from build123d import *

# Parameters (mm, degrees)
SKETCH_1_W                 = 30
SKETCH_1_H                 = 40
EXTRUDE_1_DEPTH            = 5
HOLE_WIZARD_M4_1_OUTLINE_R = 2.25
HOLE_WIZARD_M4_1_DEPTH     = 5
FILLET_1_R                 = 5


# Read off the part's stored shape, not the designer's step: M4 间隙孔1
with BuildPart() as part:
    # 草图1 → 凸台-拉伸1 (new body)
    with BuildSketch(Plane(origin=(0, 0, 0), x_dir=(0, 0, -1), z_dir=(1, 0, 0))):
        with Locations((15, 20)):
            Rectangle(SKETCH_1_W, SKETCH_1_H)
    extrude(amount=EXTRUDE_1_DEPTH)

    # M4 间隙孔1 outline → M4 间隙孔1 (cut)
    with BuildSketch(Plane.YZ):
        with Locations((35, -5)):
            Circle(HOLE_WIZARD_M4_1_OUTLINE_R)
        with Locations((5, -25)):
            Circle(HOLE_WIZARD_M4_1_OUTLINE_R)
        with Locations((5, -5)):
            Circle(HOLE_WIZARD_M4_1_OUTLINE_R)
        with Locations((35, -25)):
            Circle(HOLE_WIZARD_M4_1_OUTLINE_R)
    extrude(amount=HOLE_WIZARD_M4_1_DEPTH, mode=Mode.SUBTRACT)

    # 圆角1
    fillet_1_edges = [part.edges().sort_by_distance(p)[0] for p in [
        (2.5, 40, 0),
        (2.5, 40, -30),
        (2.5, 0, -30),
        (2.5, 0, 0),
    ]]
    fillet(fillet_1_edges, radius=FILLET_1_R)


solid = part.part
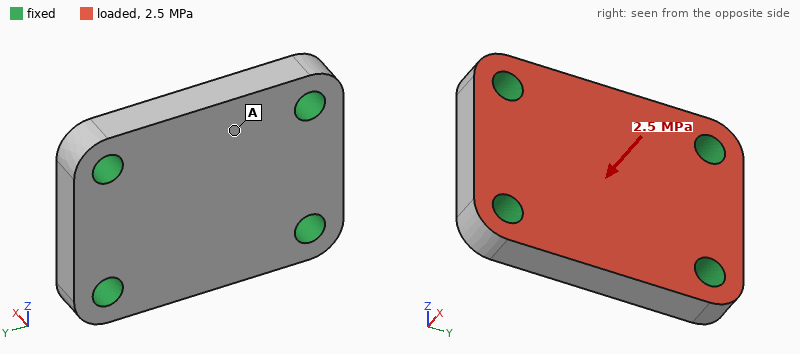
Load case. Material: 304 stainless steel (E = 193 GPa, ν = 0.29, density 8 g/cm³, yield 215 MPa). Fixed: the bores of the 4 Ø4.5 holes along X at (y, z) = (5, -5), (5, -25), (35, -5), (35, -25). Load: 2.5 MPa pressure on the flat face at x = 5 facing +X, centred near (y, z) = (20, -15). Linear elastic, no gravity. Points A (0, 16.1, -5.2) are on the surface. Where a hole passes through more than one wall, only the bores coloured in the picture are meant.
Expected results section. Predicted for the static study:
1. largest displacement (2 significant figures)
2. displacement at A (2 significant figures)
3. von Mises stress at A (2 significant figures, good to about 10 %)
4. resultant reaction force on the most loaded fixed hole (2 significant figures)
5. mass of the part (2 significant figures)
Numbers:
3.4 µm
2.7 µm
17 MPa
700 N
45 g
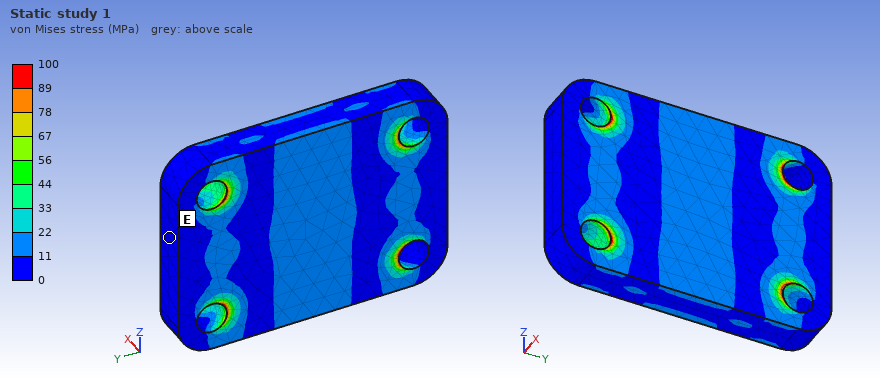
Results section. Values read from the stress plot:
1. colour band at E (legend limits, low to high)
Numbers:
0 to 11 MPa
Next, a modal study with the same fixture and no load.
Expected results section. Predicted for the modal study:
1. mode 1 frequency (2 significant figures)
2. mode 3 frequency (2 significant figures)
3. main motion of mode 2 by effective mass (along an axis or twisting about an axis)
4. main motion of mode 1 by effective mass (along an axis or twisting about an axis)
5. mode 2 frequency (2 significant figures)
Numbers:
25 kHz
43 kHz
twisting about Y
along X
31 kHz
